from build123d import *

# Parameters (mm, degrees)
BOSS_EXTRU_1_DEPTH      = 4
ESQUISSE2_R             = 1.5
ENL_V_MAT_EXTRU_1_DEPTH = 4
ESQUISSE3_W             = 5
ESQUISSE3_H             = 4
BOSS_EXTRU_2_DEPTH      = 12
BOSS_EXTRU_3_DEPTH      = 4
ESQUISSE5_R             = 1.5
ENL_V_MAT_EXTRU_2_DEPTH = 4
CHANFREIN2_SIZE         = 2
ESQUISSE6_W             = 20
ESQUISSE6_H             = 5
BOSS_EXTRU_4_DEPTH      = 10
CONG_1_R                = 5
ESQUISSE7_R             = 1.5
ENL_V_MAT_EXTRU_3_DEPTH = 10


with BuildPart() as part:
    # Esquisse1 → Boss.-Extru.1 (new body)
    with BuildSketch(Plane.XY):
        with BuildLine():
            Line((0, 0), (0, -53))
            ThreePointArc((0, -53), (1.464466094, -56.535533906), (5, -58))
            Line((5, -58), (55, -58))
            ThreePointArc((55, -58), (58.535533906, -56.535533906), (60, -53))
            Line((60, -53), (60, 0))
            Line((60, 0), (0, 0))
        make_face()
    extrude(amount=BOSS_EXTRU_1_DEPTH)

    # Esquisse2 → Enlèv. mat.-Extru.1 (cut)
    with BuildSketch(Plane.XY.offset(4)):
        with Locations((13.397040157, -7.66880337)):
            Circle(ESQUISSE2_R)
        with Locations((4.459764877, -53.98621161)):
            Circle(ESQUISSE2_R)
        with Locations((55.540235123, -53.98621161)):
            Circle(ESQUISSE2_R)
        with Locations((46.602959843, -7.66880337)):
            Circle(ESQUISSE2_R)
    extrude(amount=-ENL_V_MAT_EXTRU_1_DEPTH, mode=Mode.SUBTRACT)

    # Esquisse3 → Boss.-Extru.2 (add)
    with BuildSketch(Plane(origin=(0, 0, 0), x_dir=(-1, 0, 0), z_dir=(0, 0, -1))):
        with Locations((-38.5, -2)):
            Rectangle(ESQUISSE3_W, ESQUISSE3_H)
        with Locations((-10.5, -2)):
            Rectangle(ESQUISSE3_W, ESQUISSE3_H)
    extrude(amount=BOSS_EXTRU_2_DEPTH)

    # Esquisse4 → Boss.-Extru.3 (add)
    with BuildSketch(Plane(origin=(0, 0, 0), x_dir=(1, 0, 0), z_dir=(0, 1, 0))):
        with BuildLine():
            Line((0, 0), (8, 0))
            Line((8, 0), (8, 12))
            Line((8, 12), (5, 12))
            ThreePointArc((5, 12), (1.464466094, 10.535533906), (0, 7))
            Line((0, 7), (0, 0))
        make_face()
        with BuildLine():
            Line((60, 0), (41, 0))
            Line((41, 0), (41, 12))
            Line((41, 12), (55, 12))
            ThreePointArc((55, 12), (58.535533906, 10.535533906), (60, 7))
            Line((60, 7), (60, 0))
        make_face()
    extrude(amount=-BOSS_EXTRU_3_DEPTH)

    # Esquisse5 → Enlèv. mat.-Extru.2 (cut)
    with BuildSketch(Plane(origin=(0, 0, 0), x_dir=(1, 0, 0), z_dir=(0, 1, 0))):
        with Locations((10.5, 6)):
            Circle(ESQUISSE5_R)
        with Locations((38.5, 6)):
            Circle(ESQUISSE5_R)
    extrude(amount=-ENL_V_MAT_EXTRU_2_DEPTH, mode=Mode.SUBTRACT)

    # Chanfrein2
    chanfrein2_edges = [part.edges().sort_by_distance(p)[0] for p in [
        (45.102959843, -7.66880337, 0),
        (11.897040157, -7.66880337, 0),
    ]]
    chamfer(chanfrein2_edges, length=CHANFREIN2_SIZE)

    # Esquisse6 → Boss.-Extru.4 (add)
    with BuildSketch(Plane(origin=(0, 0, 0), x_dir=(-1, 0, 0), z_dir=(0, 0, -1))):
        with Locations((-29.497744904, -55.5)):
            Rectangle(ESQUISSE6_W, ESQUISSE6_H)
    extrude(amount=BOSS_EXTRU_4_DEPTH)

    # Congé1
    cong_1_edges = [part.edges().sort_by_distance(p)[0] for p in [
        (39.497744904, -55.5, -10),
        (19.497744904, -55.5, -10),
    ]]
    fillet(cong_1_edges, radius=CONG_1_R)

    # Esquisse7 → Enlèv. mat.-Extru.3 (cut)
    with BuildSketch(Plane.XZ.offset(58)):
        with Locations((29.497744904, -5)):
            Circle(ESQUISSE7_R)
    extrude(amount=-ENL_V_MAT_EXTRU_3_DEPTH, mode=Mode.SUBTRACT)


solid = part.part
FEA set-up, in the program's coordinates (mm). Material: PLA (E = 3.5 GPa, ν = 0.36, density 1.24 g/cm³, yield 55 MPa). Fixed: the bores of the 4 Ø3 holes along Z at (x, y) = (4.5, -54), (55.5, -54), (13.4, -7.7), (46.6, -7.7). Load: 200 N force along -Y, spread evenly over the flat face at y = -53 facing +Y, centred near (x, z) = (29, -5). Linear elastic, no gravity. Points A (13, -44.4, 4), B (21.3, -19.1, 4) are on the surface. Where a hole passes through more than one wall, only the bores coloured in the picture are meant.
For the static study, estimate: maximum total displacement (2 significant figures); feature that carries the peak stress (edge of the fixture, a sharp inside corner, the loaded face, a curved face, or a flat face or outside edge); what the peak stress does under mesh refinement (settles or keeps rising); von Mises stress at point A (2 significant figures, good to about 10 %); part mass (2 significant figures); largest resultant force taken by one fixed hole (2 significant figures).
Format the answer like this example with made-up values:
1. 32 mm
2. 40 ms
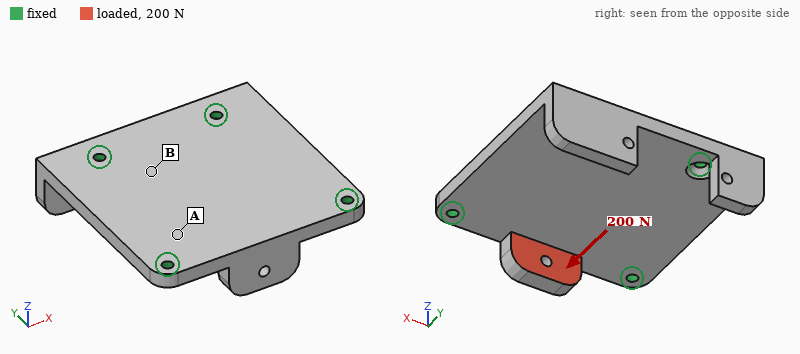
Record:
1. 0.36 mm
2. edge of the fixture
3. keeps rising
4. 3.2 MPa
5. 20 g
6. 67 N
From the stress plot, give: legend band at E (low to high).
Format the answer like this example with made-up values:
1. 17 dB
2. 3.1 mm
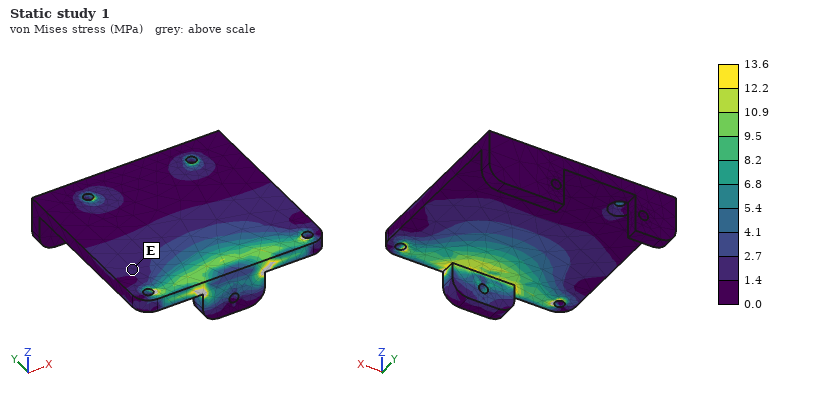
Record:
1. 1.4 to 2.7 MPa
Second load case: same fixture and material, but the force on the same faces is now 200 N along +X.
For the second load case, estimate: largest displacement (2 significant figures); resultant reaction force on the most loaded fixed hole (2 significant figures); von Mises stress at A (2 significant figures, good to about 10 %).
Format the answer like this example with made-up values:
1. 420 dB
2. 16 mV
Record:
1. 0.11 mm
2. 96 N
3. 1.6 MPa
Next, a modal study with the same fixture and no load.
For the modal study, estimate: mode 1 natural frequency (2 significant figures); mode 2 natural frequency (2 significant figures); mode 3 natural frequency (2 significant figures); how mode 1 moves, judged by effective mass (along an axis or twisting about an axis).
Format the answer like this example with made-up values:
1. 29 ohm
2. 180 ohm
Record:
1. 1900 Hz
2. 2400 Hz
3. 2600 Hz
4. along Z
